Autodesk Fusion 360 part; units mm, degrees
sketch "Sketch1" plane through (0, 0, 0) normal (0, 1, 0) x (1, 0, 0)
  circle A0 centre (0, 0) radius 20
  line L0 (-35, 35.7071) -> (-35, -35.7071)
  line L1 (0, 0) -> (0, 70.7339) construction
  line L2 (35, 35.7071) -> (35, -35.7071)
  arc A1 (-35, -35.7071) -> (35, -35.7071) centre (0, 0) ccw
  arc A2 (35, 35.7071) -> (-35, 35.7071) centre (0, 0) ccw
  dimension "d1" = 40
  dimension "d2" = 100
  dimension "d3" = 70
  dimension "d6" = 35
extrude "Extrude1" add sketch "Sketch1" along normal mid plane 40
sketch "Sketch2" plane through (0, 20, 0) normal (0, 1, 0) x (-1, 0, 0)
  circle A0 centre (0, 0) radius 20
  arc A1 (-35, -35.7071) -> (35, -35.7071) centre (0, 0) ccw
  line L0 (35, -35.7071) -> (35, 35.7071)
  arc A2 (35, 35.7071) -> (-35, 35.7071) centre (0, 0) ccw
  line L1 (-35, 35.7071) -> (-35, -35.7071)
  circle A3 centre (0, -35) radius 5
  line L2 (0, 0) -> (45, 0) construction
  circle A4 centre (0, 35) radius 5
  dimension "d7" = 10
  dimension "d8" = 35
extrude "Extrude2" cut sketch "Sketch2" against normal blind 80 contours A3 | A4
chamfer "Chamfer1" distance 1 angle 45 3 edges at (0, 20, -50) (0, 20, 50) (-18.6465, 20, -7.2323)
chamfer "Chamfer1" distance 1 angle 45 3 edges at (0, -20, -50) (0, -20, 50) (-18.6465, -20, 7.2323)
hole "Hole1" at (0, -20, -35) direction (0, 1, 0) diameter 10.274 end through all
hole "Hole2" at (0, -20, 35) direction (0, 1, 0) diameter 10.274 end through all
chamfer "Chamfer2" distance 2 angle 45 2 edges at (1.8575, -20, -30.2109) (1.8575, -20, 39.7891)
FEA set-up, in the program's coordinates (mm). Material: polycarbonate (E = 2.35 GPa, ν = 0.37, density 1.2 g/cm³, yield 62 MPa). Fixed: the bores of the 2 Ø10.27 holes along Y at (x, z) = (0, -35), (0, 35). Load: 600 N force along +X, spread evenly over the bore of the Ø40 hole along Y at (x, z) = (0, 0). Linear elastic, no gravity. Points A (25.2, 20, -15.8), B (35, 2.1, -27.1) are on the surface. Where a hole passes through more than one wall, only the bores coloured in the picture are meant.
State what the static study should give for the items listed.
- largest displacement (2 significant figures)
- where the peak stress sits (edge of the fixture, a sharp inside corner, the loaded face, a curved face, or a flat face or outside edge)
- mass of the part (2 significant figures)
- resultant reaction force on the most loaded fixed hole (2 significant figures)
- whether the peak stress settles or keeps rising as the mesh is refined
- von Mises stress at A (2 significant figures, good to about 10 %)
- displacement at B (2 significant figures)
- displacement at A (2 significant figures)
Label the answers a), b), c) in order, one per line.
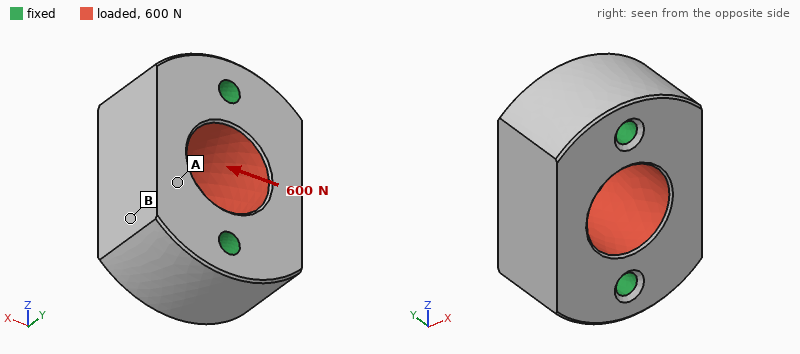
a) 6.1 µm
b) edge of the fixture
c) 240 g
d) 300 N
e) keeps rising
f) 0.20 MPa
g) 2.9 µm
h) 3.8 µm
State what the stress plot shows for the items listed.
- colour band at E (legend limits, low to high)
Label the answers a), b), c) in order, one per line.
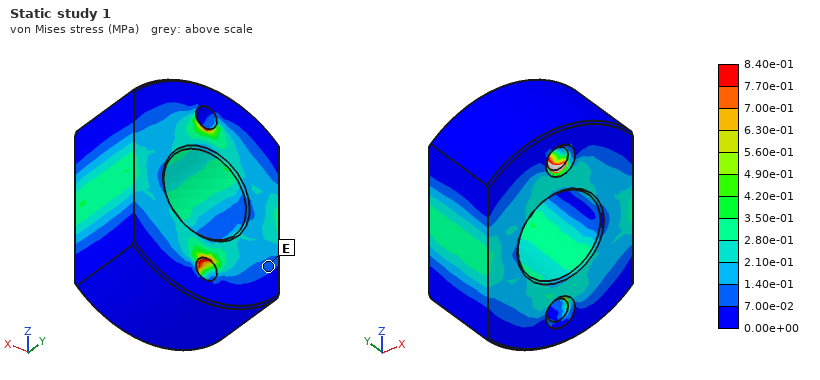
a) 7.00e-02 to 1.40e-01 MPa
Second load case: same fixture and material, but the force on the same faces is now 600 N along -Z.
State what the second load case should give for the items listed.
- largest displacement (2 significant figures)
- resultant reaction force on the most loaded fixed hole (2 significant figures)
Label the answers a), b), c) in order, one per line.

a) 4.5 µm
b) 300 N
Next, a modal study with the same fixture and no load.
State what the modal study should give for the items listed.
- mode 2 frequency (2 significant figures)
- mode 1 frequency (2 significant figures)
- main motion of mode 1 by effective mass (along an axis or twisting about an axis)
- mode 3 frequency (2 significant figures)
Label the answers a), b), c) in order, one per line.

a) 3600 Hz
b) 3300 Hz
c) twisting about Z
d) 3700 Hz
